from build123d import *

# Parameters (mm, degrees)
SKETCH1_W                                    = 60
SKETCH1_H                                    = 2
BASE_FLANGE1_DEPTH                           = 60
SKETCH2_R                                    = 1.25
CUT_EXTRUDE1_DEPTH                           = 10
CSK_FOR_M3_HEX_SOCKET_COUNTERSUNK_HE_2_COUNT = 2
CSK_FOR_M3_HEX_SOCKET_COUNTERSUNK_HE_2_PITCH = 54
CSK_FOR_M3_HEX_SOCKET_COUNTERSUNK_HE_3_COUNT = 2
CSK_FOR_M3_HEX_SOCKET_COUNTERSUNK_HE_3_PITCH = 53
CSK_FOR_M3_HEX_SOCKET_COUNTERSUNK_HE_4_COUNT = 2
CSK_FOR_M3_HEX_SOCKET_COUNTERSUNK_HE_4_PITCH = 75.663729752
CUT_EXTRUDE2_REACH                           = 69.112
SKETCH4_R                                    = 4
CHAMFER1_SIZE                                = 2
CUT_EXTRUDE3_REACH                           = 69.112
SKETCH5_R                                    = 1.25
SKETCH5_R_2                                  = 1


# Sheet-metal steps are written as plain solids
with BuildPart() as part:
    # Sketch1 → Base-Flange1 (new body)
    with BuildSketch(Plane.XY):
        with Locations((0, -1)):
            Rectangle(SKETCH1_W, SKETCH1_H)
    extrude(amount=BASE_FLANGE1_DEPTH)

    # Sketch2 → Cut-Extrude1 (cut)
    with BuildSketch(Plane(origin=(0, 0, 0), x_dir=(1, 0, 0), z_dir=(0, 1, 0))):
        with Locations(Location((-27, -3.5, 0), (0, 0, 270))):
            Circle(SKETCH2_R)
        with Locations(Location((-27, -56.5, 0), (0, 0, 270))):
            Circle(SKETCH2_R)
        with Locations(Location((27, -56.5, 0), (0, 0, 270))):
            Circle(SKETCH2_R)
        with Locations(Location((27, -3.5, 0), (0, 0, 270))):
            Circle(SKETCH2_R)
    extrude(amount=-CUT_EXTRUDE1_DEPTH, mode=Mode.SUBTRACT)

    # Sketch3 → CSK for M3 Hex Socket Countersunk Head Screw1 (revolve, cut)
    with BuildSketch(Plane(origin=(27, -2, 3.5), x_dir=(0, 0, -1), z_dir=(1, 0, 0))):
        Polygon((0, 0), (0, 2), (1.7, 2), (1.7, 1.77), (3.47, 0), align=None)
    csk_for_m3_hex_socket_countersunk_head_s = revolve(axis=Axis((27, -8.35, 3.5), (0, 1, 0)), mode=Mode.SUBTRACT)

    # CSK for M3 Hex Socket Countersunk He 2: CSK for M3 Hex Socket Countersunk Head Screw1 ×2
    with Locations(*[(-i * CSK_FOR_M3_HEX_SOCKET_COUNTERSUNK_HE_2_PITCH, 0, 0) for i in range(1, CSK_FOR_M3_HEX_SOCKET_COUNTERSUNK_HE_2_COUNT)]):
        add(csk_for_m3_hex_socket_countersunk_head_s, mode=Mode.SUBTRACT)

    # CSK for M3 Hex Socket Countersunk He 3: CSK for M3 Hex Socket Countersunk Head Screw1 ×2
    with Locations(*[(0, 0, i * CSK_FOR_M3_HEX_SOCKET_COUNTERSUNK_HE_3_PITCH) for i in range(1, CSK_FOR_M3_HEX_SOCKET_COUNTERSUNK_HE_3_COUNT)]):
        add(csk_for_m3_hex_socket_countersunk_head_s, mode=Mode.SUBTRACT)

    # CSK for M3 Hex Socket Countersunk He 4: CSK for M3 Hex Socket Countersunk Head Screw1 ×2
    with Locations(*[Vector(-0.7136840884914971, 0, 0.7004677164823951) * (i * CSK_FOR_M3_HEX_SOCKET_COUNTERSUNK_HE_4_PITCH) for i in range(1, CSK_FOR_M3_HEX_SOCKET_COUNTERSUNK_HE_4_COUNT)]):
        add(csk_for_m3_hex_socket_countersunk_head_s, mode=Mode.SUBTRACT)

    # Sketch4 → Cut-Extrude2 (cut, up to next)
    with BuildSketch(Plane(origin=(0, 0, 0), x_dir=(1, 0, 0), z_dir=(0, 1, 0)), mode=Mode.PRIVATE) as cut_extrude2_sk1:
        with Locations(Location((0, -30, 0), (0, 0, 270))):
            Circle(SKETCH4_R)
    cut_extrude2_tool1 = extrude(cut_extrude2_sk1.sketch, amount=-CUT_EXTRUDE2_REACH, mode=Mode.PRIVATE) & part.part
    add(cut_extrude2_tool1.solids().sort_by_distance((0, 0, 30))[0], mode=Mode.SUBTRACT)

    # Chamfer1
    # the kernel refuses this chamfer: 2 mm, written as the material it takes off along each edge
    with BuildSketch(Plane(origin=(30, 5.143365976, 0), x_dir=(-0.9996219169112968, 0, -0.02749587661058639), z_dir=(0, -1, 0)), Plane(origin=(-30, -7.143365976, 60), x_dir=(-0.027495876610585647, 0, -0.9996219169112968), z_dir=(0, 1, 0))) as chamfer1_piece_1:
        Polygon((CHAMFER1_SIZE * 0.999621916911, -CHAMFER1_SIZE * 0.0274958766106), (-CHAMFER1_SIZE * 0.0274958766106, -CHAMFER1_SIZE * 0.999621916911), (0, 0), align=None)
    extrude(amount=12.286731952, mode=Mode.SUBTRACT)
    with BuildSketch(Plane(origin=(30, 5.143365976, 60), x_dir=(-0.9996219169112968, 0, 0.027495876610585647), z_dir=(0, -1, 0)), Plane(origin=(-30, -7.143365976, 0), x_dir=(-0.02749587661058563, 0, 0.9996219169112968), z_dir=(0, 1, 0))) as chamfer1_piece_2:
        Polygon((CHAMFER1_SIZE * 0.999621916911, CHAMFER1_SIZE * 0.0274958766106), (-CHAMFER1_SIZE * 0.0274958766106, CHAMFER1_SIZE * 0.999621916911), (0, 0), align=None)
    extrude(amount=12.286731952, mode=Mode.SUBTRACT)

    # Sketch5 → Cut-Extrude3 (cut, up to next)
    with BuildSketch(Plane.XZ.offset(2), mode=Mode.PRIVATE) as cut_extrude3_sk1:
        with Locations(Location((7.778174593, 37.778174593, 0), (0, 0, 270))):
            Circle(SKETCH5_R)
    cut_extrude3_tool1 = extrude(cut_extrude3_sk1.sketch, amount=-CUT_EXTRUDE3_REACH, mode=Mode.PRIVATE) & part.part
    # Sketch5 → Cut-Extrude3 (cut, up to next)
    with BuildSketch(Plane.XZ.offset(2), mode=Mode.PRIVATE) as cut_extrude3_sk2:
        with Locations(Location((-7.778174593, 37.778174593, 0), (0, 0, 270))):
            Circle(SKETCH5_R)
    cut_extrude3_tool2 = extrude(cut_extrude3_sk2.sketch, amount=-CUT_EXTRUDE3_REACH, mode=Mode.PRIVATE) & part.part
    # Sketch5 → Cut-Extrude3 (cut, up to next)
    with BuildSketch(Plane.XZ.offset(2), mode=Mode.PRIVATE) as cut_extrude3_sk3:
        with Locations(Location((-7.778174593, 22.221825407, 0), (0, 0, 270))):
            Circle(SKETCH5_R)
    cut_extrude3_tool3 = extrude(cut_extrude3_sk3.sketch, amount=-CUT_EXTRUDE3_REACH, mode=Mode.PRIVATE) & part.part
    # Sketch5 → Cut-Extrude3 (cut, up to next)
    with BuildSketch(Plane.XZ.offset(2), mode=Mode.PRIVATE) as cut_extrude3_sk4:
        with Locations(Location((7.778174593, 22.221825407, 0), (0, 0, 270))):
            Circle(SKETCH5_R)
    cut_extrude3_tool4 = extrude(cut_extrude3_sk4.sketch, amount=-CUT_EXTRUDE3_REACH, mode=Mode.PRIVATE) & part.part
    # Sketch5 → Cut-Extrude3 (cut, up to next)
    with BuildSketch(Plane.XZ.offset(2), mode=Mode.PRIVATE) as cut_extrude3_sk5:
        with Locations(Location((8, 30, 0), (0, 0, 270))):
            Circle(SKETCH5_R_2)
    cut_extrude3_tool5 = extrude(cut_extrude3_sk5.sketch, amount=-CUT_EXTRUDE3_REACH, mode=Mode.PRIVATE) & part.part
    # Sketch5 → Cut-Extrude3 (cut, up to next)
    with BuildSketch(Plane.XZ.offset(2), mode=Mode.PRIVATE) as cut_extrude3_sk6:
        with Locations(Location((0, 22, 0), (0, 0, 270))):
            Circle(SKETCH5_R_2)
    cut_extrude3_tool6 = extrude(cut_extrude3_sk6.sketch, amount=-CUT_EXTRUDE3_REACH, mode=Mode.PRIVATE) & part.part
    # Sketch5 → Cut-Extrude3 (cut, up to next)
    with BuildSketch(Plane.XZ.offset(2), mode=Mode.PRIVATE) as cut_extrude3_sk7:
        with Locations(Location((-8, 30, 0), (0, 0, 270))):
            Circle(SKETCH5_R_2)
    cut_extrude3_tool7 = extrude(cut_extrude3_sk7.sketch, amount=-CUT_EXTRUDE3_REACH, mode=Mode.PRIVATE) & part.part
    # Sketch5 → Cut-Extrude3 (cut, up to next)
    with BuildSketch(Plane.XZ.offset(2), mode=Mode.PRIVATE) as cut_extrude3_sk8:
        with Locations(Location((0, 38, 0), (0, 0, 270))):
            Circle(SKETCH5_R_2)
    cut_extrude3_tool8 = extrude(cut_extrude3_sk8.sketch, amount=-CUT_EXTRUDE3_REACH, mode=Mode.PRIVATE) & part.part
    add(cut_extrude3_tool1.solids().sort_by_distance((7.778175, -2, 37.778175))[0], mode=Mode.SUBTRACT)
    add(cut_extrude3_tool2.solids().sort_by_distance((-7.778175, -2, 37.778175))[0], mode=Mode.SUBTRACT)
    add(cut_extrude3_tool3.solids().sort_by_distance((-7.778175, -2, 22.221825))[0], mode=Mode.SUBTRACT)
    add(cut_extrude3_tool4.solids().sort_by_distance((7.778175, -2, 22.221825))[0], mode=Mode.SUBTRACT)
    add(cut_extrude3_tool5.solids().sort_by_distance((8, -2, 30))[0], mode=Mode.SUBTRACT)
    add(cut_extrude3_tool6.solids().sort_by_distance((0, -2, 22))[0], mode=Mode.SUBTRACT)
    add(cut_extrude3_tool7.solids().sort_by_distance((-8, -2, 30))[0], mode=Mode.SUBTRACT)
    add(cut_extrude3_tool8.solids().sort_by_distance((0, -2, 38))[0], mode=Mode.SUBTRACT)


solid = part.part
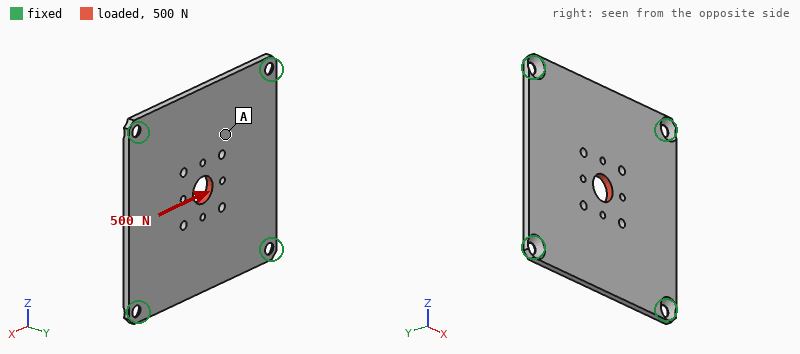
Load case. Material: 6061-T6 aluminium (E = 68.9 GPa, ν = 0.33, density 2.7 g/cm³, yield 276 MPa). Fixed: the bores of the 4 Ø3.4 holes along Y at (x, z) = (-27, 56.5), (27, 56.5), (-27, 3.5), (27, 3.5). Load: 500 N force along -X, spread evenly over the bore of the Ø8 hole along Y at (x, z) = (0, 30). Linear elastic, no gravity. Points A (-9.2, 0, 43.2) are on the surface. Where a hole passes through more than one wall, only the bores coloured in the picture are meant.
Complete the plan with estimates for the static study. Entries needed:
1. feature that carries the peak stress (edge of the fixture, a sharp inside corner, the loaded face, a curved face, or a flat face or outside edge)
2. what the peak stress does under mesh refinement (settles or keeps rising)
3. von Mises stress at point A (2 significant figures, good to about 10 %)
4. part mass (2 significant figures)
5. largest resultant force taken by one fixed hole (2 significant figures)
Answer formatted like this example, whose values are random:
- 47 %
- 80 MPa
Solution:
- edge of the fixture
- keeps rising
- 5.3 MPa
- 19 g
- 130 N
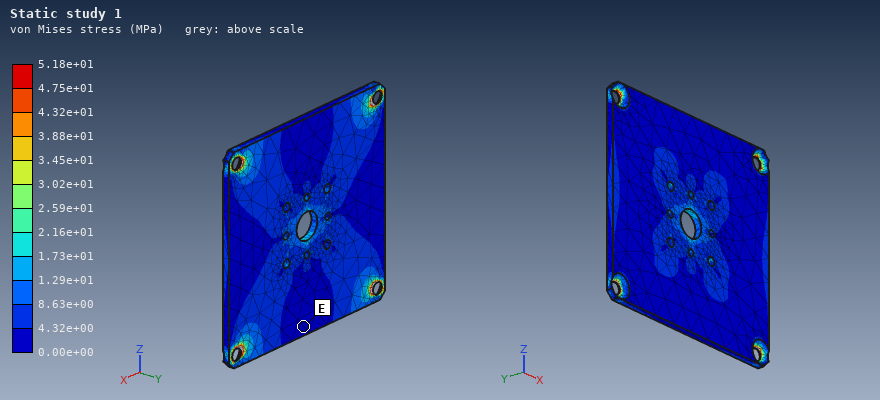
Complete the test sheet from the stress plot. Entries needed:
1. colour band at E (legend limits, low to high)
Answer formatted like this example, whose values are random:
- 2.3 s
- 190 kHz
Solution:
- 0.00e+00 to 4.32e+00 MPa
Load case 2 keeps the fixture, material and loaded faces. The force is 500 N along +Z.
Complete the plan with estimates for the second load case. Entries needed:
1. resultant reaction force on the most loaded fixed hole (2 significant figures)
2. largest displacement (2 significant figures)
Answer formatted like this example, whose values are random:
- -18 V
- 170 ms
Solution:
- 130 N
- 6.0 µm
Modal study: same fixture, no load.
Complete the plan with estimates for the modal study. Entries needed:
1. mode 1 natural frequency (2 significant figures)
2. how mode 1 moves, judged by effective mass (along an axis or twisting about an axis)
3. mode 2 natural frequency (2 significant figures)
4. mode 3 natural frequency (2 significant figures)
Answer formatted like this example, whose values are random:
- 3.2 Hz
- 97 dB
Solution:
- 1900 Hz
- along Y
- 3400 Hz
- 3500 Hz
